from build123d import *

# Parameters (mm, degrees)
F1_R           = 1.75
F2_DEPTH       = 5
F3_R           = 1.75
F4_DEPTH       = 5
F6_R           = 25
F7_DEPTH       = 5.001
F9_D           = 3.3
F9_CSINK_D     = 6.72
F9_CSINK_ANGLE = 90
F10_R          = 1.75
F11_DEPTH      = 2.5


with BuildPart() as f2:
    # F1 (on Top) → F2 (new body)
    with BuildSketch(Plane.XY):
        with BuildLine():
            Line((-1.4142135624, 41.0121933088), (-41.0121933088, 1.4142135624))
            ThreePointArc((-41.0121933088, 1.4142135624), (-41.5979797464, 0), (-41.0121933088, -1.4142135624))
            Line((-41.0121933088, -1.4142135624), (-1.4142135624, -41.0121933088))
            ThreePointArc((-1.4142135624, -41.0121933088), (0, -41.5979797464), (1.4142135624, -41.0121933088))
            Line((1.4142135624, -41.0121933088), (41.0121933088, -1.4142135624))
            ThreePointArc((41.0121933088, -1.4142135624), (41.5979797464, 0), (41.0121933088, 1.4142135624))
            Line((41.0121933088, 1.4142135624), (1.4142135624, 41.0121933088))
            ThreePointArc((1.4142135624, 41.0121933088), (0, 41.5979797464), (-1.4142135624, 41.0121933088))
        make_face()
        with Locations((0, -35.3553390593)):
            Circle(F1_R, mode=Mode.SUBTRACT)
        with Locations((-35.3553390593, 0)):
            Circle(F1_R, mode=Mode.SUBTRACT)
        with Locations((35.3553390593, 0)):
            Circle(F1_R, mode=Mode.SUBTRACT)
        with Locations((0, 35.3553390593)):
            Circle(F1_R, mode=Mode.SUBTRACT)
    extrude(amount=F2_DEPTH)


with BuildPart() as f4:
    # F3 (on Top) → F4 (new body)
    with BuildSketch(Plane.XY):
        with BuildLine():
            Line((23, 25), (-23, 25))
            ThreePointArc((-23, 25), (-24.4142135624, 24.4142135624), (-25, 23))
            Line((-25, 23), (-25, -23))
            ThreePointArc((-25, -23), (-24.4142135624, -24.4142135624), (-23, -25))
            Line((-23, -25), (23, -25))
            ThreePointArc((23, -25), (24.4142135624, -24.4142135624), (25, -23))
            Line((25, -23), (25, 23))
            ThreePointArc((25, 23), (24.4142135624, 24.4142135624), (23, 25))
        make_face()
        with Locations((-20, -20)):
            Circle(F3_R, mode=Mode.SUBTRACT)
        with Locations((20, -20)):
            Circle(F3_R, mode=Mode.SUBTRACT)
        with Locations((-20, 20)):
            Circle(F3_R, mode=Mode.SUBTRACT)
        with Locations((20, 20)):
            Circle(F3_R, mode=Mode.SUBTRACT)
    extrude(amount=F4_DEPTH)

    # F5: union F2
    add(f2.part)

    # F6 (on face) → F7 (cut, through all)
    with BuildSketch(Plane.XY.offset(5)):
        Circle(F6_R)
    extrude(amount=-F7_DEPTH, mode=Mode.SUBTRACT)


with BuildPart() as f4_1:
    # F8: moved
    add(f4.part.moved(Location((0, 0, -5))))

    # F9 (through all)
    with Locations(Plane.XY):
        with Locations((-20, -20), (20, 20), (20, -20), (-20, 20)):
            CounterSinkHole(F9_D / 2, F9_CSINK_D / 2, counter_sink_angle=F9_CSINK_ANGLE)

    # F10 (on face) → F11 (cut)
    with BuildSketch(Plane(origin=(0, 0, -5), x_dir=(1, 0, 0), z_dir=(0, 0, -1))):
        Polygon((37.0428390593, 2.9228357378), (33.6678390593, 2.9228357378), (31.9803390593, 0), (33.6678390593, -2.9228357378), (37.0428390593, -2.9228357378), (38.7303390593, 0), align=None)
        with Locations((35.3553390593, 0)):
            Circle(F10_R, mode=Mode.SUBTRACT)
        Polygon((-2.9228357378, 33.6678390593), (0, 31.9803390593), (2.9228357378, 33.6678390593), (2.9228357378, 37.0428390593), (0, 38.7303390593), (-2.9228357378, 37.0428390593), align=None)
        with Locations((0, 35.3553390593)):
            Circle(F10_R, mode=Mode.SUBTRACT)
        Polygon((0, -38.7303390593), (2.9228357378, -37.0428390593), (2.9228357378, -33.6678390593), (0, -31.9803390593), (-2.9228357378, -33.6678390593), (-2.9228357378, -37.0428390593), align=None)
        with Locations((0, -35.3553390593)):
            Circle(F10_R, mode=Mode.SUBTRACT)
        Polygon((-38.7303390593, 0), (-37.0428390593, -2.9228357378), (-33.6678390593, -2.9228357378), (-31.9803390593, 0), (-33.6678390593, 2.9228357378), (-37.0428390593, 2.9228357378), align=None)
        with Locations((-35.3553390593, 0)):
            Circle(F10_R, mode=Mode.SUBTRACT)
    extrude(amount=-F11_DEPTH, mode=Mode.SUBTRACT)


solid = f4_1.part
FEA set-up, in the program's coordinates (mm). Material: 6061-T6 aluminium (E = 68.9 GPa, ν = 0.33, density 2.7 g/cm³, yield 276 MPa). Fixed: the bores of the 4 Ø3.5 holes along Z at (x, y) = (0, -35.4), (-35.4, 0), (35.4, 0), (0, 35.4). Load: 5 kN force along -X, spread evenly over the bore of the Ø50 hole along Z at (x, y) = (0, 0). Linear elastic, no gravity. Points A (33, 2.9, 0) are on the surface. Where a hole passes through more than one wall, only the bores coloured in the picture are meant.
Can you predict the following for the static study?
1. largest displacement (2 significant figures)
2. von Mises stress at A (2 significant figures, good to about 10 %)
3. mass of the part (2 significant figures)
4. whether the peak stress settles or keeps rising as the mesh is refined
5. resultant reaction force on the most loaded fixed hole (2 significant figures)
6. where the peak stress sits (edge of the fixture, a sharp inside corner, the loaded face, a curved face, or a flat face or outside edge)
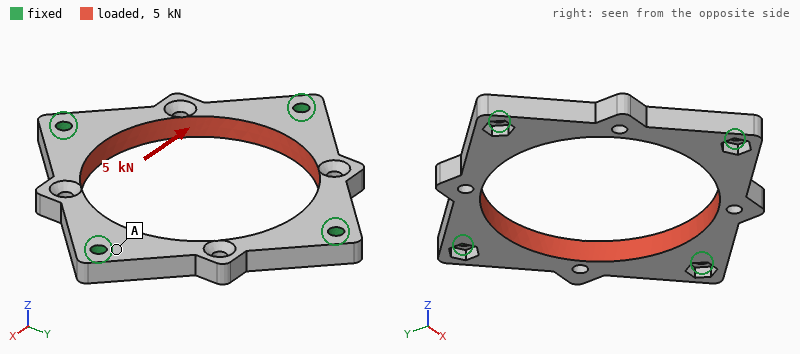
35 µm
27 MPa
22 g
keeps rising
1.4 kN
edge of the fixture
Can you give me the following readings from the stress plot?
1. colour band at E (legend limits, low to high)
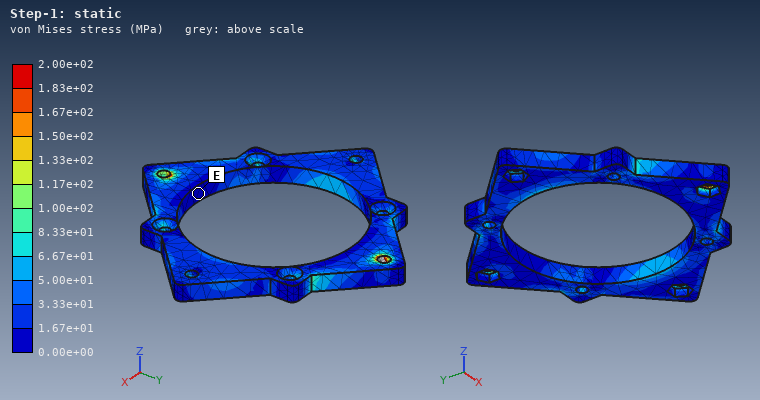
0.00e+00 to 1.67e+01 MPa
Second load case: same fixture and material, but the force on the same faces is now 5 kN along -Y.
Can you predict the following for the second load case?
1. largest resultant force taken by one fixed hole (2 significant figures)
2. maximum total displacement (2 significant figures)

1.4 kN
35 µm
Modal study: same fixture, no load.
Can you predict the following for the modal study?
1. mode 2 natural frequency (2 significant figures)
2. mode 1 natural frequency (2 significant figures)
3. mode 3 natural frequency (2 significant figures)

8600 Hz
7500 Hz
8600 Hz
